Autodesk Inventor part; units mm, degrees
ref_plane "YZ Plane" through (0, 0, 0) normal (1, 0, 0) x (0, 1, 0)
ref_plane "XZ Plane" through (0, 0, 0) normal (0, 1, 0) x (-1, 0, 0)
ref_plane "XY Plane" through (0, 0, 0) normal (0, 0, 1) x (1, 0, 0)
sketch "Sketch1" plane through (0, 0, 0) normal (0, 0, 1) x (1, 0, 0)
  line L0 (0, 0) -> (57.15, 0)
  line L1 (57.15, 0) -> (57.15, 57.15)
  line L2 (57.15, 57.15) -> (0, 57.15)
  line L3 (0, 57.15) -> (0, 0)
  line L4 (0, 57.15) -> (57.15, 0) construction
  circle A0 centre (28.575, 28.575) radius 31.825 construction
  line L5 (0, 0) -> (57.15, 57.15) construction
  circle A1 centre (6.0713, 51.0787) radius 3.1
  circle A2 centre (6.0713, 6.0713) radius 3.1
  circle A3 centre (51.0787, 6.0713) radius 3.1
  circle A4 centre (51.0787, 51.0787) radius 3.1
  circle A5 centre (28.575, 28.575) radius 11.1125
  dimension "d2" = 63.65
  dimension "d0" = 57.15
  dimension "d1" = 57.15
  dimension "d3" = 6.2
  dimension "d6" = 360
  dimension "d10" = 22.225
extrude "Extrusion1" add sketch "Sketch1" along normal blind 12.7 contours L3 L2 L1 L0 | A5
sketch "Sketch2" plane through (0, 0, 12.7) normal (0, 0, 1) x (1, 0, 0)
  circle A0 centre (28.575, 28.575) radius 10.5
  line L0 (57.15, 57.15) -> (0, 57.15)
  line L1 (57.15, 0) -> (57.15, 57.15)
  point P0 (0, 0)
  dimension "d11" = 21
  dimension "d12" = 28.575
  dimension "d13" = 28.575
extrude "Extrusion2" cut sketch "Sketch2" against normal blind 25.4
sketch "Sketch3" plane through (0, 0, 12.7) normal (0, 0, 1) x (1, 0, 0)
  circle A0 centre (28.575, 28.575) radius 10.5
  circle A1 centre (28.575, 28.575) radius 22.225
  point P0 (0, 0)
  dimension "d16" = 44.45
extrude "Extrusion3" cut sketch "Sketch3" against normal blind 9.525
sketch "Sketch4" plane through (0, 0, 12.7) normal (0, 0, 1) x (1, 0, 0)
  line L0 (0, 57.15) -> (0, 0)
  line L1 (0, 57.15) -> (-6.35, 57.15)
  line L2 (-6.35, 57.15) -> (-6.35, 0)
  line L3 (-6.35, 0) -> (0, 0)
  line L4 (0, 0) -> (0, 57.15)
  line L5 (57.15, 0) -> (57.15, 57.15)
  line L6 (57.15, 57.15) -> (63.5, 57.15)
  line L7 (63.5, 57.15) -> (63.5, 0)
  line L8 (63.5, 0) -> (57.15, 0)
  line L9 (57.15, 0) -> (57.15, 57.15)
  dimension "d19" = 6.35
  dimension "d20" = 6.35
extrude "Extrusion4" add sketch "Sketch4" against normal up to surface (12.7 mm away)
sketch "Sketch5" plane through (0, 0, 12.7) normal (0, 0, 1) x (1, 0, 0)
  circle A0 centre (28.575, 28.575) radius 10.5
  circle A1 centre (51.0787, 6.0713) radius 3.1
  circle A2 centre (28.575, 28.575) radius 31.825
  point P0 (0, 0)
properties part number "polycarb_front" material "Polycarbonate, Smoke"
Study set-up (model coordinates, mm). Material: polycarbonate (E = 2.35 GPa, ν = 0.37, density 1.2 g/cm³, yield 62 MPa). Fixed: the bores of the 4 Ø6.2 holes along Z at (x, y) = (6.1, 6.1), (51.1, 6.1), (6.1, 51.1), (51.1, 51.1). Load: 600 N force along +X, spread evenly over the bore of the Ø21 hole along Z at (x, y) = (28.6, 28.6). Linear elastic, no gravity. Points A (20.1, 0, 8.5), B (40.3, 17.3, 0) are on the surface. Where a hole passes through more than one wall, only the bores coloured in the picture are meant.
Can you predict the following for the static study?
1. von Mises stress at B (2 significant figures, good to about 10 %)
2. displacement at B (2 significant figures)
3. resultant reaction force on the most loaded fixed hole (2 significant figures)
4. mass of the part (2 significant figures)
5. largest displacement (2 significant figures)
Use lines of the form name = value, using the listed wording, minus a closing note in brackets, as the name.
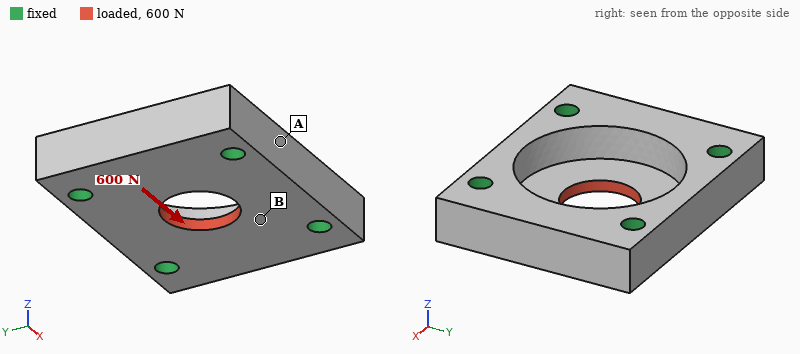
von Mises stress at B = 2.3 MPa
displacement at B = 18 µm
resultant reaction force on the most loaded fixed hole = 150 N
mass of the part = 40 g
largest displacement = 33 µm
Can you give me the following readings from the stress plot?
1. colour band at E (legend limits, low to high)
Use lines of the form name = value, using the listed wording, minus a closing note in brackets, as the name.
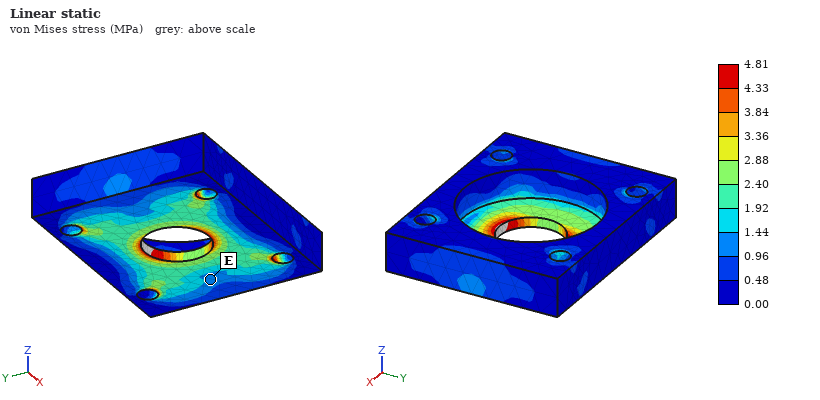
colour band at E = 0.96 to 1.44 MPa
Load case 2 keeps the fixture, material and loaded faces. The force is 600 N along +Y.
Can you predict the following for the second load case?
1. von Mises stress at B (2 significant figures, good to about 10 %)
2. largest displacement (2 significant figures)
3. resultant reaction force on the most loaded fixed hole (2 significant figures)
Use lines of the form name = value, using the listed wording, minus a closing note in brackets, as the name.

von Mises stress at B = 2.5 MPa
largest displacement = 40 µm
resultant reaction force on the most loaded fixed hole = 160 N
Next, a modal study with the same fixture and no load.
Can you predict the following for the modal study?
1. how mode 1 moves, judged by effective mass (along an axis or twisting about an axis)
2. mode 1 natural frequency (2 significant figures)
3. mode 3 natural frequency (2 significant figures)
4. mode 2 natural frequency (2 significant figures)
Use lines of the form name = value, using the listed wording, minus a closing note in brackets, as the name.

how mode 1 moves, judged by effective mass = along Z
mode 1 natural frequency = 4800 Hz
mode 3 natural frequency = 6000 Hz
mode 2 natural frequency = 6000 Hz
